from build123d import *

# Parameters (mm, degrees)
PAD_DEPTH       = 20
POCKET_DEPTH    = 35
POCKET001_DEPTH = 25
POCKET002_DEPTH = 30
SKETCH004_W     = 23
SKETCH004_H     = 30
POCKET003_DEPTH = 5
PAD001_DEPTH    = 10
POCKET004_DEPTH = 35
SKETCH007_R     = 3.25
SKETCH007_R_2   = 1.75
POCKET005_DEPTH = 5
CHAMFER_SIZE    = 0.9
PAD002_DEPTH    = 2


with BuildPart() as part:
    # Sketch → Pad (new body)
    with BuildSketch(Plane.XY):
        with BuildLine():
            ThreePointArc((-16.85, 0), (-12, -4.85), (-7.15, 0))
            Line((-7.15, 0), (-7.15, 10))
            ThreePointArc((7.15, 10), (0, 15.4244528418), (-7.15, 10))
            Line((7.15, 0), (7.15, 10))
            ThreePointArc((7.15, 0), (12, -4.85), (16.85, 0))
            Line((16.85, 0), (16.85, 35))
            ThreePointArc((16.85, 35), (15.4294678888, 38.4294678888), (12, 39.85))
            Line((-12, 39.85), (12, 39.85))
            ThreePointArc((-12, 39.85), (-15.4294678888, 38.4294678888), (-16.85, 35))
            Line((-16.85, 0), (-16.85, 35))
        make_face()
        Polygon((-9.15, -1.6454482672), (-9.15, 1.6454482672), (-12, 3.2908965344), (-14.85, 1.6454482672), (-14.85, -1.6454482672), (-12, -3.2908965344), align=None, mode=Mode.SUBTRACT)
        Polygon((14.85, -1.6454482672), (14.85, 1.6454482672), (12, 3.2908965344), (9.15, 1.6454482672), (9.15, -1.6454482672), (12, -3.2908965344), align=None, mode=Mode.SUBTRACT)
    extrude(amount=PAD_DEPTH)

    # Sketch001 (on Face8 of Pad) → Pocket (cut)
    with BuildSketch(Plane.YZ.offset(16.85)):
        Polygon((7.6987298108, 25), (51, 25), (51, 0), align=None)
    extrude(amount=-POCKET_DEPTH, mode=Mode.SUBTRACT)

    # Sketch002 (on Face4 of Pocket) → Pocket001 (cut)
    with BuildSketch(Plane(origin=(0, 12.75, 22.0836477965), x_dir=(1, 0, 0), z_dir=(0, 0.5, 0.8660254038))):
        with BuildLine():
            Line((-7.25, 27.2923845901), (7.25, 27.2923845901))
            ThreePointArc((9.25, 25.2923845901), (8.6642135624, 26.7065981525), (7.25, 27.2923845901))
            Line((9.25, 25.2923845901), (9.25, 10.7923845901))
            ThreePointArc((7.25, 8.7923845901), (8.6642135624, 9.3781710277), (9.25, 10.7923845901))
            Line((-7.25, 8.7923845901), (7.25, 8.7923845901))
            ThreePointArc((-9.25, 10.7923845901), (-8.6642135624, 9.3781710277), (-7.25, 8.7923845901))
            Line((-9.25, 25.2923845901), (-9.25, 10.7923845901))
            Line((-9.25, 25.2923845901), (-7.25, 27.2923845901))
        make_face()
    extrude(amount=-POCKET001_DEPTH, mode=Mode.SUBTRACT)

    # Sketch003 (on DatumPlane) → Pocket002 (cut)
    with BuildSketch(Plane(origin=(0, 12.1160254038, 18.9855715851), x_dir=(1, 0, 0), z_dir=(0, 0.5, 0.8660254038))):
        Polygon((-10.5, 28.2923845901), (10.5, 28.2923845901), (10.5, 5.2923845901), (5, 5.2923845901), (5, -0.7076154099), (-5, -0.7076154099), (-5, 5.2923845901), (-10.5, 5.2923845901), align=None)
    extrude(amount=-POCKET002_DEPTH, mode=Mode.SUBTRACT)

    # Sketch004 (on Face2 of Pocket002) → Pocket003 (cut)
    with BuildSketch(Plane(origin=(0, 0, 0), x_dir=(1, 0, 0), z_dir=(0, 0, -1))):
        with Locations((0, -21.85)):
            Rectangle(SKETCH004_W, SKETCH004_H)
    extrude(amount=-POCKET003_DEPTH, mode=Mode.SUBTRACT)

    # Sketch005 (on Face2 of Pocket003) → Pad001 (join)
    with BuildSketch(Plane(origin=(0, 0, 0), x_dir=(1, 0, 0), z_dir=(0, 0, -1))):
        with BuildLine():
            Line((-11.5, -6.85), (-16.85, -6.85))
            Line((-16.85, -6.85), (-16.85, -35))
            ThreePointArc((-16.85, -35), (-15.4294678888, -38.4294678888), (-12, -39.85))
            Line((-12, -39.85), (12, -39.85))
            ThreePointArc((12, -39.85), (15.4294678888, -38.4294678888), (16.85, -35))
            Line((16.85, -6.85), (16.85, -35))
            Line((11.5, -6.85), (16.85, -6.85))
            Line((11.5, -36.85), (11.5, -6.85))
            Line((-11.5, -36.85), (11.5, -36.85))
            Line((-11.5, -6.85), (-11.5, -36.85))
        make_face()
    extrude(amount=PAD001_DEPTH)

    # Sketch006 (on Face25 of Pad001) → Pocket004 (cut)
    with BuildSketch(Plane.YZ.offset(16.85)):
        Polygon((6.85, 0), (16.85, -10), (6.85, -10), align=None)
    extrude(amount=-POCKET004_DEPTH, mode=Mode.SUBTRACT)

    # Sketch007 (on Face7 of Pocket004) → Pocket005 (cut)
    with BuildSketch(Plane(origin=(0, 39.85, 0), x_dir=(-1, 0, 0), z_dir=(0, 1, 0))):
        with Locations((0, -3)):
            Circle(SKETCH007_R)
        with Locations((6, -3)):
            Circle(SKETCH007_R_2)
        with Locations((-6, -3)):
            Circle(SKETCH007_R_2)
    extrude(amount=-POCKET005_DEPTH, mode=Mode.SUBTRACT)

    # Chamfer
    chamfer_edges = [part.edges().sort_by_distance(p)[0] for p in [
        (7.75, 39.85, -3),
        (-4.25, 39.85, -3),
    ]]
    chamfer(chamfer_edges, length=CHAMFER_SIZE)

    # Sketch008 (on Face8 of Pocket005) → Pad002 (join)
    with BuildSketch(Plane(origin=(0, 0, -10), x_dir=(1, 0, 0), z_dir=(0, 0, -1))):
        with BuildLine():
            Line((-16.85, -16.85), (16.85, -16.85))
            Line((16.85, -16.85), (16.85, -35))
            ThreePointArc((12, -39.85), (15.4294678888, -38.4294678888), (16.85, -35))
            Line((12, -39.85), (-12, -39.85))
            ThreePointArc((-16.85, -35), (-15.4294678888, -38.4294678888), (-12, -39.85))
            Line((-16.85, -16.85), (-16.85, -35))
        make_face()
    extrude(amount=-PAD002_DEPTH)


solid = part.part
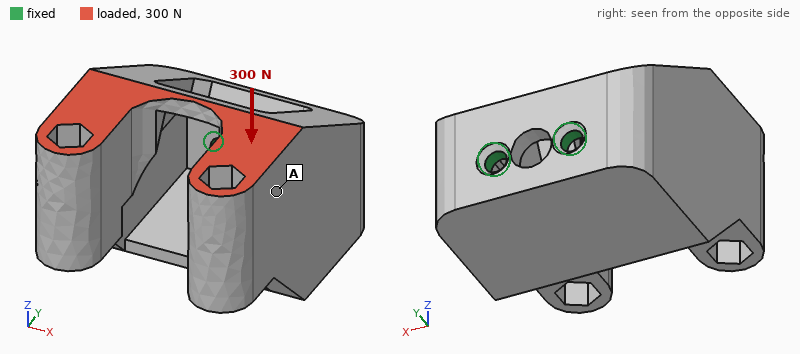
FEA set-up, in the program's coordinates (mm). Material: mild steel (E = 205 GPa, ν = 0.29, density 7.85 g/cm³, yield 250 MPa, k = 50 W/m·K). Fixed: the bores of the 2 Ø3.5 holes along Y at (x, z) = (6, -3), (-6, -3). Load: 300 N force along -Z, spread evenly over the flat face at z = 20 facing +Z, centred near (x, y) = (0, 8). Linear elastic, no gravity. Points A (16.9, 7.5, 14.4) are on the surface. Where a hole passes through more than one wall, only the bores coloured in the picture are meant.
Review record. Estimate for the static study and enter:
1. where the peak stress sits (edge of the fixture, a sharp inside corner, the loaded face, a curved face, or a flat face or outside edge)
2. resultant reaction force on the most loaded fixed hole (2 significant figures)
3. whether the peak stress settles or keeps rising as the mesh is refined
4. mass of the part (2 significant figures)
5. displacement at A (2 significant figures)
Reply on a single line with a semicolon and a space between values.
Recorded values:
edge of the fixture; 160 N; keeps rising; 120 g; 64 µm
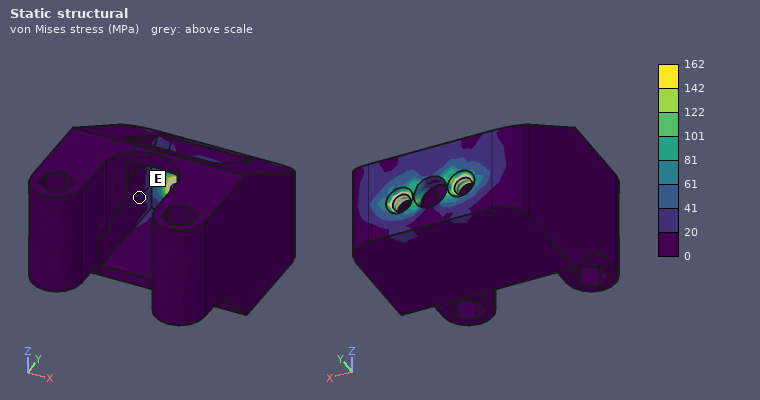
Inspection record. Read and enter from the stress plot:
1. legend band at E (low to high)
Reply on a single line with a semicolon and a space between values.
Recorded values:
0 to 20 MPa
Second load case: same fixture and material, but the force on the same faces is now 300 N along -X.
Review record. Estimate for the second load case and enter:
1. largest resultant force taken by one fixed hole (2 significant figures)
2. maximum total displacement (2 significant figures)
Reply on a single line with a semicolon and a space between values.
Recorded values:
680 N; 38 µm
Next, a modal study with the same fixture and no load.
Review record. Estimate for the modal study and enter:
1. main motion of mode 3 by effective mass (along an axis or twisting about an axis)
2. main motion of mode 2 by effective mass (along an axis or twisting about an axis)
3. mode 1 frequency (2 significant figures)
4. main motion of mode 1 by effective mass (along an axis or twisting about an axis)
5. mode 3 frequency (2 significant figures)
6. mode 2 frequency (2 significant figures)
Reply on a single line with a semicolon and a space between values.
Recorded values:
twisting about Y; along X; 1300 Hz; along Z; 3700 Hz; 2200 Hz
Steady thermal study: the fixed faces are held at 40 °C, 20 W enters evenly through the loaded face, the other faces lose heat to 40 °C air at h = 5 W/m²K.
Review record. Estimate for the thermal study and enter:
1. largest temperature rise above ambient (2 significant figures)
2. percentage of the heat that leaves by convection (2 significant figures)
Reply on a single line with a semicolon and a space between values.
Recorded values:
75 K; 9.5 %
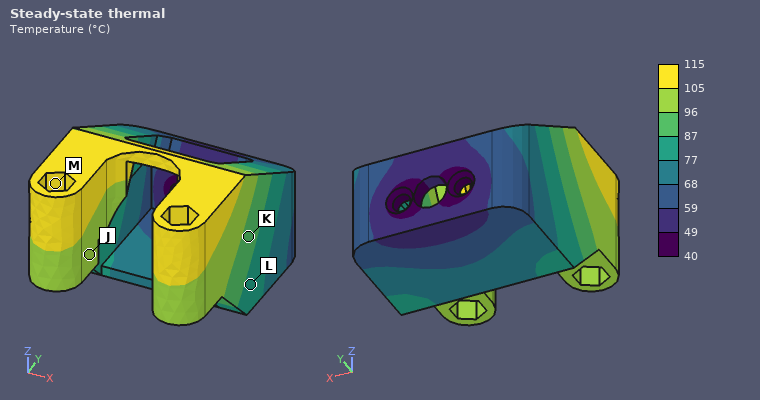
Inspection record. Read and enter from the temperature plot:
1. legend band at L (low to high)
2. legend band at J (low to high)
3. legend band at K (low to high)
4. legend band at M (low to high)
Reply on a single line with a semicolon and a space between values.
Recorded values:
77 to 87 °C; 96 to 105 °C; 87 to 96 °C; 105 to 115 °C
